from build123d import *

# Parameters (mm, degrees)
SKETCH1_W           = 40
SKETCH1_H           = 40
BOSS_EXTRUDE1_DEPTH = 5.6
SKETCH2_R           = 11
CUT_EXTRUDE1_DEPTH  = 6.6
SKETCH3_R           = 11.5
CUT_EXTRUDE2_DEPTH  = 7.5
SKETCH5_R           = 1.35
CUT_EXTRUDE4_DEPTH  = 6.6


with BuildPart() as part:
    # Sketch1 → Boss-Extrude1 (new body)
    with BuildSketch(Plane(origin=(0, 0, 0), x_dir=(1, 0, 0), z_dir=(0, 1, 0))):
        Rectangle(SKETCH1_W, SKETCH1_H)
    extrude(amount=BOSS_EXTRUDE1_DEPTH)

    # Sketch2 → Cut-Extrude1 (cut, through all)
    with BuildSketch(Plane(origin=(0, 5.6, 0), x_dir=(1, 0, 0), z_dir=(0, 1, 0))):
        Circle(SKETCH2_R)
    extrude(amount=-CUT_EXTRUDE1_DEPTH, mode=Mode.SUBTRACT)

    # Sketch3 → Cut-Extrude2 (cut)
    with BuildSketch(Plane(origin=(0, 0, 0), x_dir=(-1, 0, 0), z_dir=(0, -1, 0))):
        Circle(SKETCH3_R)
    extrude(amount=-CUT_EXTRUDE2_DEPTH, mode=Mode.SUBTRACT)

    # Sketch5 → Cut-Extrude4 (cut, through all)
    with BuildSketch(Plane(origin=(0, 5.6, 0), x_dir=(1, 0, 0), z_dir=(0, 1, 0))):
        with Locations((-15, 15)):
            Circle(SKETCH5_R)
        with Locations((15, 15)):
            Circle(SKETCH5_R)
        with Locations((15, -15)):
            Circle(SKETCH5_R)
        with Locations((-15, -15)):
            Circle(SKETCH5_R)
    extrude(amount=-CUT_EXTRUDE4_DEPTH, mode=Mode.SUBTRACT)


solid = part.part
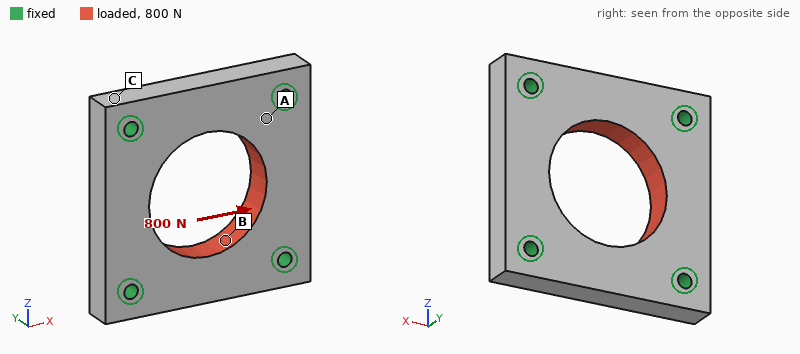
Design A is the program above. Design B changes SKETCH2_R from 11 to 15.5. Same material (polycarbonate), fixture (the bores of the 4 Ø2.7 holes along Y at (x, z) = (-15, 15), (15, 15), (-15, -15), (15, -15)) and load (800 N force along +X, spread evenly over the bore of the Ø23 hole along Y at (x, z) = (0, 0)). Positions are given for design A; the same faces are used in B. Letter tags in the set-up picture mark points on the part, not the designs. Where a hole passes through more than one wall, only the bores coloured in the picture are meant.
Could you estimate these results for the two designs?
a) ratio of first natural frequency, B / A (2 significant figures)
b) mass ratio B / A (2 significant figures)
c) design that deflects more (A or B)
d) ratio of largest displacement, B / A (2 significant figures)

1.1
0.71
B
1.7
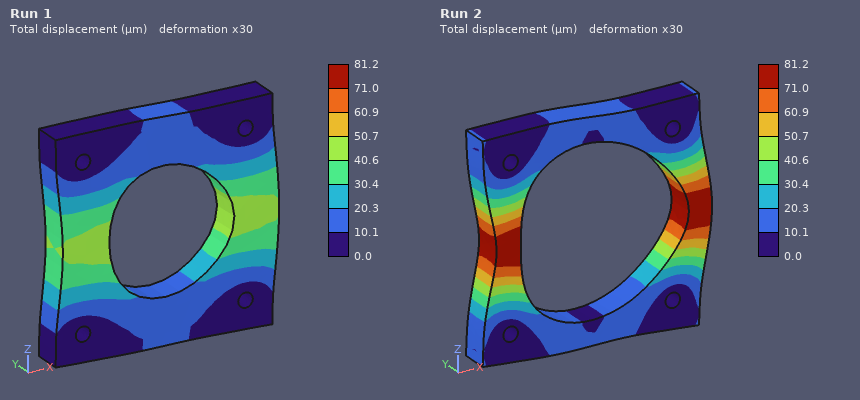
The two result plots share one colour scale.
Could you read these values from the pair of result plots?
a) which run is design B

Run 2
